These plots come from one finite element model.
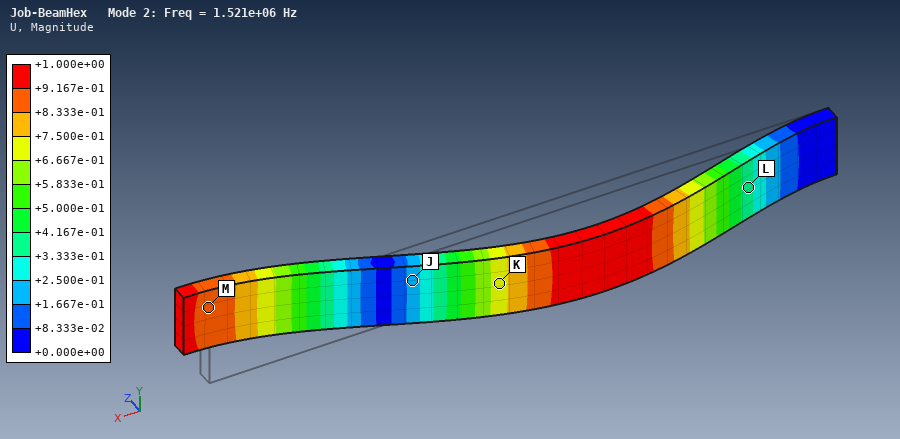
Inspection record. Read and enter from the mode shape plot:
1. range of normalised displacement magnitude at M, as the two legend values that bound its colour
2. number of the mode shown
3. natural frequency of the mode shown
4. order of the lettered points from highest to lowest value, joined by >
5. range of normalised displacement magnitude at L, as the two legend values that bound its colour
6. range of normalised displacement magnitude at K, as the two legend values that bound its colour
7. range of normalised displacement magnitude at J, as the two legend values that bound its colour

+8.333e-01 to +9.167e-01
2
1.521e+06 Hz
M > K > L > J
+3.333e-01 to +4.167e-01
+6.667e-01 to +7.500e-01
+1.667e-01 to +2.500e-01
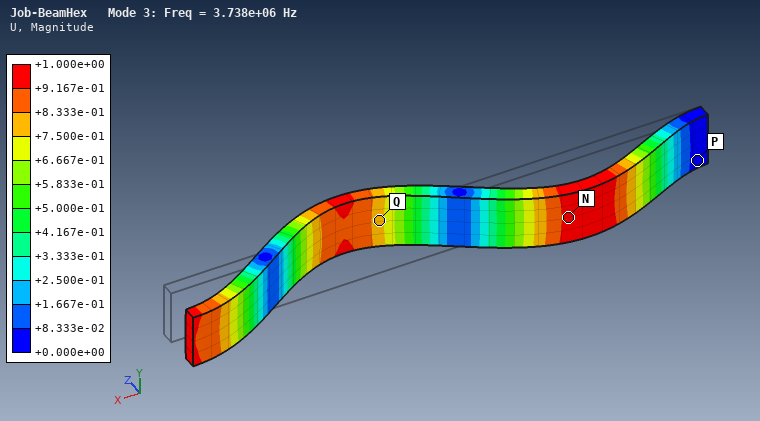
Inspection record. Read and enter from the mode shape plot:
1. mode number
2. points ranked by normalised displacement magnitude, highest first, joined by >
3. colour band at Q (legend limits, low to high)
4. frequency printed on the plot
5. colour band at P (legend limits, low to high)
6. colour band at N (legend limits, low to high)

3
N > Q > P
+7.500e-01 to +8.333e-01
3.738e+06 Hz
+0.000e+00 to +8.333e-02
+9.167e-01 to +1.000e+00
